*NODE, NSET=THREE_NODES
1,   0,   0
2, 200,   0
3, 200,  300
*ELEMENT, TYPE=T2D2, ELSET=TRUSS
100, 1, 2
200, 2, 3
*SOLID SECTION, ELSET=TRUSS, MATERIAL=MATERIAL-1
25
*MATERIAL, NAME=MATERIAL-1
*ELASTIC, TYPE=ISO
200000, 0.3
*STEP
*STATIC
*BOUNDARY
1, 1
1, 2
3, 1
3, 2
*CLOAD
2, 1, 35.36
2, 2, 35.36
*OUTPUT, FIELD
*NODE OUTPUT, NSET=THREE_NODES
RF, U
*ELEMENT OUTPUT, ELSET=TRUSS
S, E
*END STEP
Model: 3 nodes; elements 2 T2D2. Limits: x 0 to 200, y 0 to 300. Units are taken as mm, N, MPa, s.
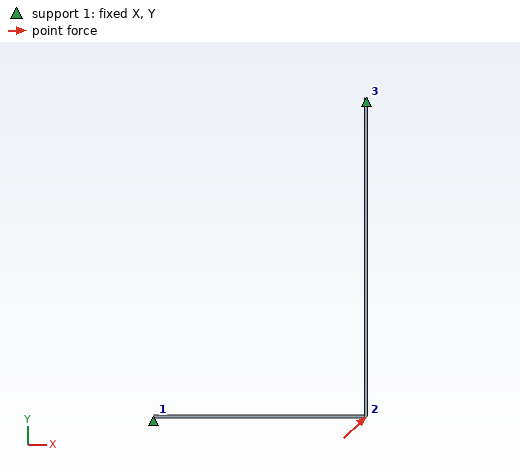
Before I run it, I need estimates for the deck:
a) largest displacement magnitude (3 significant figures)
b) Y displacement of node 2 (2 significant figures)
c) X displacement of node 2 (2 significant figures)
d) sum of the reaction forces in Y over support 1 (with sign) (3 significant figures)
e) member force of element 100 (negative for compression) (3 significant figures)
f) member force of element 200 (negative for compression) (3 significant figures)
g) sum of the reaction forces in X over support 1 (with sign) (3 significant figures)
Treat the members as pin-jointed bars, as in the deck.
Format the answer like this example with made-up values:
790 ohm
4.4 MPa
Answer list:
0.00255 mm
0.0021 mm
0.0014 mm
-35.4 N
35.4 N
-35.4 N
-35.4 N
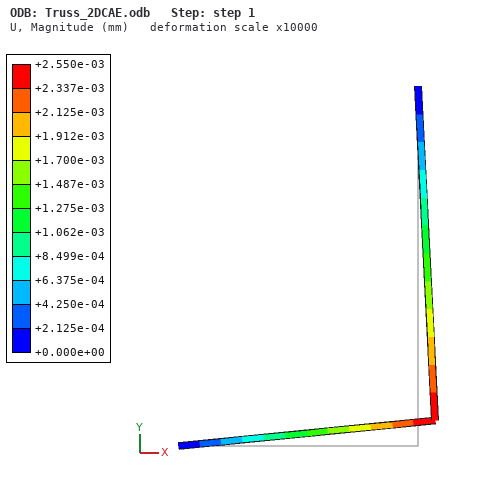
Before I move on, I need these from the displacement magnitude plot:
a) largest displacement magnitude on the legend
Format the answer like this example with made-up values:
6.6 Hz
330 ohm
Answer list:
+2.550e-03 mm
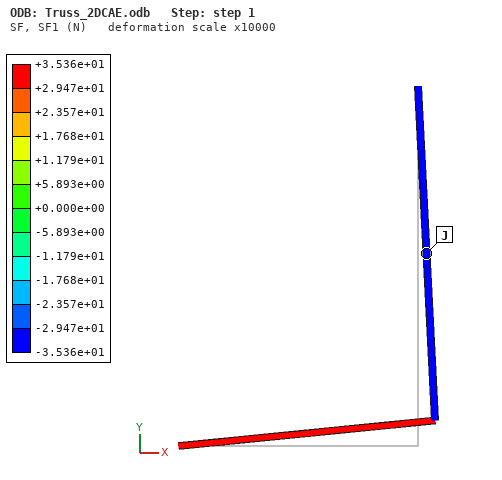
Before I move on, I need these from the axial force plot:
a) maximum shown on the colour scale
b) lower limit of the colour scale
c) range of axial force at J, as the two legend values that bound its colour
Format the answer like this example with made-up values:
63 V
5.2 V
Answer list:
+3.536e+01 N
-3.536e+01 N
-3.536e+01 to -2.947e+01 N
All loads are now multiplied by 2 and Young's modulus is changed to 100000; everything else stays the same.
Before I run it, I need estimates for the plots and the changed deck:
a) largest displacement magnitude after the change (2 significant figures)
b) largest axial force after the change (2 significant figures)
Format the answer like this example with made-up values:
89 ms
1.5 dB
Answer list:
0.010 mm
71 N
